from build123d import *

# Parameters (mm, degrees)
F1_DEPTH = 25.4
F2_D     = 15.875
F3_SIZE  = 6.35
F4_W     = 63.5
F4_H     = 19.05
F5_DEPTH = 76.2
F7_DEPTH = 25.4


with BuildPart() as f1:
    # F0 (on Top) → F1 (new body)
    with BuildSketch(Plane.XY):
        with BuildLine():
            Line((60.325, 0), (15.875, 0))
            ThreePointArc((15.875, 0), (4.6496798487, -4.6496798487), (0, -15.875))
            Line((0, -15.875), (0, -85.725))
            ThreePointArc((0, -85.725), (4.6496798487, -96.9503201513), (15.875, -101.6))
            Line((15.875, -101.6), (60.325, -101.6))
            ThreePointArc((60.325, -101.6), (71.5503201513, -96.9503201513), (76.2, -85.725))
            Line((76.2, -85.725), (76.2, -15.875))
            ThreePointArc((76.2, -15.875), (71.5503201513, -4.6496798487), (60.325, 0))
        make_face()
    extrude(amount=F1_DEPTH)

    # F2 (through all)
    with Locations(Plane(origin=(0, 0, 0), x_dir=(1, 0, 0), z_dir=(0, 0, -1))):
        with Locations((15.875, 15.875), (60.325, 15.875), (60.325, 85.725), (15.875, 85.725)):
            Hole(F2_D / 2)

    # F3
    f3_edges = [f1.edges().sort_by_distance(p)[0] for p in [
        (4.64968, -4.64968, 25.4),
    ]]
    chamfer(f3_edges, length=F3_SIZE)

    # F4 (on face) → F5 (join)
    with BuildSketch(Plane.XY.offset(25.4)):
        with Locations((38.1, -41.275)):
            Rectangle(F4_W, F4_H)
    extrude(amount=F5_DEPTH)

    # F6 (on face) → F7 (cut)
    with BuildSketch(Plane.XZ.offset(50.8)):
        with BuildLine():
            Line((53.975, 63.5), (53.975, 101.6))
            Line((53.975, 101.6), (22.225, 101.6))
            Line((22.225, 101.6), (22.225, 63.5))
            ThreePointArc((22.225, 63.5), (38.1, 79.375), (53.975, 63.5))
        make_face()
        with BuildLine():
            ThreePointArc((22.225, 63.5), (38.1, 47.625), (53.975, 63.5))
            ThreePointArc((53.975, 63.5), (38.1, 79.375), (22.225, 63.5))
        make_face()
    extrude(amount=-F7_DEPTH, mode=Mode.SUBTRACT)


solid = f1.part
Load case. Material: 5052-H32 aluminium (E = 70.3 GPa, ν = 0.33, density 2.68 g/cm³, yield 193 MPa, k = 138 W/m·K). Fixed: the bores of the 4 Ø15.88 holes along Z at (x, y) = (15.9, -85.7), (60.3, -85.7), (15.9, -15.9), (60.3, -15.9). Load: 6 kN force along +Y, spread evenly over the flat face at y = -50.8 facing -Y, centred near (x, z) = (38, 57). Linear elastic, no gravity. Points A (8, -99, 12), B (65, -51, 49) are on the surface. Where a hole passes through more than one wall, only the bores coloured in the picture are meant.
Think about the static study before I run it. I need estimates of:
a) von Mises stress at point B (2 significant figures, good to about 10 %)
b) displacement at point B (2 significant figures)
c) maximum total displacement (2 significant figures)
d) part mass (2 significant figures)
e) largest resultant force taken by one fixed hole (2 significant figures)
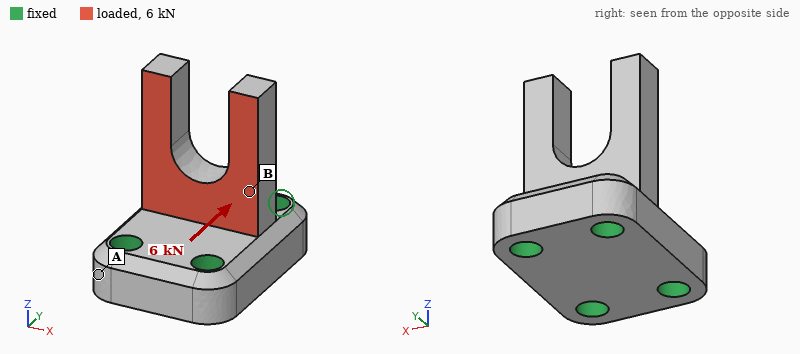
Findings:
33 MPa
0.041 mm
0.18 mm
610 g
3.1 kN
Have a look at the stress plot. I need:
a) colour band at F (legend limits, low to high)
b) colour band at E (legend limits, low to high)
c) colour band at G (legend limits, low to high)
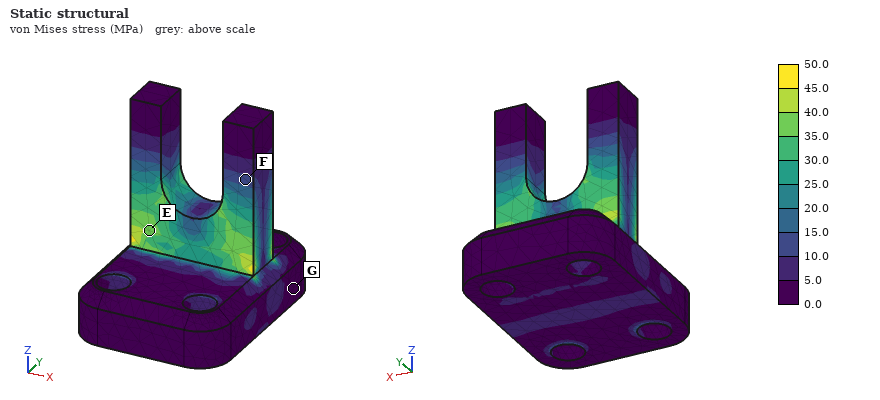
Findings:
10.0 to 15.0 MPa
35.0 to 40.0 MPa
0.0 to 5.0 MPa
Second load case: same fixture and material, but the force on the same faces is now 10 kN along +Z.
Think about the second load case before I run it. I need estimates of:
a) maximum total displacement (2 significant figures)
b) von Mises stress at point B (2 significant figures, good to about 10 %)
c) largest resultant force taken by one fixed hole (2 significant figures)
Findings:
0.11 mm
30 MPa
2.6 kN
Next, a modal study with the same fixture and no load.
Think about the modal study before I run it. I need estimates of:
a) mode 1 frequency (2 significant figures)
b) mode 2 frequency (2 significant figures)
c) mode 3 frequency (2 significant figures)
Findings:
2900 Hz
3200 Hz
3700 Hz
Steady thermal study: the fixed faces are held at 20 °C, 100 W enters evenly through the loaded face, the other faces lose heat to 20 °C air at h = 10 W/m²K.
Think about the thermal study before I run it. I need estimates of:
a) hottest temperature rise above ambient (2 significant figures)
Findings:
35 K
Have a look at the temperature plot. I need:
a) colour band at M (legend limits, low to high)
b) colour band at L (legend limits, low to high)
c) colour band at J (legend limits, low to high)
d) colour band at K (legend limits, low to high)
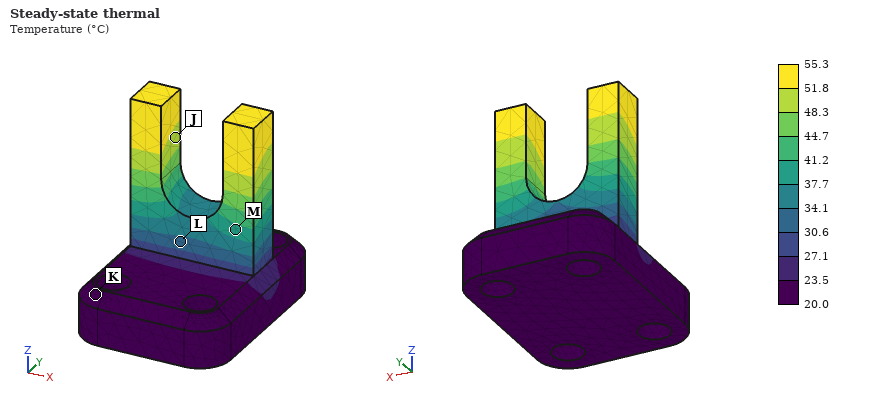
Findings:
37.7 to 41.2 °C
30.6 to 34.1 °C
48.3 to 51.8 °C
20.0 to 23.5 °C
